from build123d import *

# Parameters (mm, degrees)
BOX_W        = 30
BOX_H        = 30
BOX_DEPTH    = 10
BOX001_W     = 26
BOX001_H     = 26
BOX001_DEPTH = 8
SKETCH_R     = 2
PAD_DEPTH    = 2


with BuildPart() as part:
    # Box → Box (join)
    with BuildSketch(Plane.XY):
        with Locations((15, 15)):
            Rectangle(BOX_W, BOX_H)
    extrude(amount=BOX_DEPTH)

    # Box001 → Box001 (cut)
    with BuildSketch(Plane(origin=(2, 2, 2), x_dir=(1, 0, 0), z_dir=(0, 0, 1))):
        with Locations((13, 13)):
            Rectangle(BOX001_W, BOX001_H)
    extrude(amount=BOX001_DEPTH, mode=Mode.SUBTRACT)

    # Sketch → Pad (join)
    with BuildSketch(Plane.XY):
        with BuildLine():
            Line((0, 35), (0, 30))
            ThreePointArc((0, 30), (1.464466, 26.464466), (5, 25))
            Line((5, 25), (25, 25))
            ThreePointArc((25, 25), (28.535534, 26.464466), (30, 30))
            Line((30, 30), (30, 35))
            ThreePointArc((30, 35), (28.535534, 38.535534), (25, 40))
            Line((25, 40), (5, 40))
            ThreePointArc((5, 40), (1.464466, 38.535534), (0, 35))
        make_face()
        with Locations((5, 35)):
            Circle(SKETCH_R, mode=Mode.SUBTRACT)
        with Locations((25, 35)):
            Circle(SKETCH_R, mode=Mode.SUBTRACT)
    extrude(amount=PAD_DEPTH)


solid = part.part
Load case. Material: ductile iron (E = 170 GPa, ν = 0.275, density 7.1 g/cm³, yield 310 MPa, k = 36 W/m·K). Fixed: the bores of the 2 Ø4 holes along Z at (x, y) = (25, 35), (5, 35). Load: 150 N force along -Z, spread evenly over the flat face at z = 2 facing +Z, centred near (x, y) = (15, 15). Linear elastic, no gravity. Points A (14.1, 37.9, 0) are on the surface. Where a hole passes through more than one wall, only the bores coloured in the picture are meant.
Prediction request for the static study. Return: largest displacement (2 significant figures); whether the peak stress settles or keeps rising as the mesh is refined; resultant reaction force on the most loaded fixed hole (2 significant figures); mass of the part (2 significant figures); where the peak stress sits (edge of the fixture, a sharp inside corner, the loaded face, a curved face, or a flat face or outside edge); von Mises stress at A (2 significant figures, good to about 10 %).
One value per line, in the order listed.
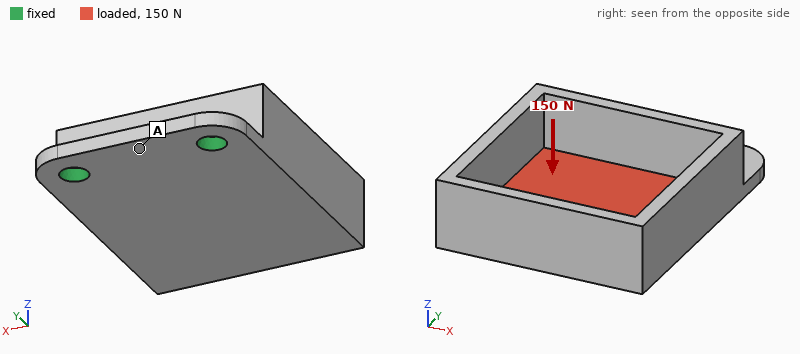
0.14 mm
keeps rising
82 N
29 g
edge of the fixture
20 MPa
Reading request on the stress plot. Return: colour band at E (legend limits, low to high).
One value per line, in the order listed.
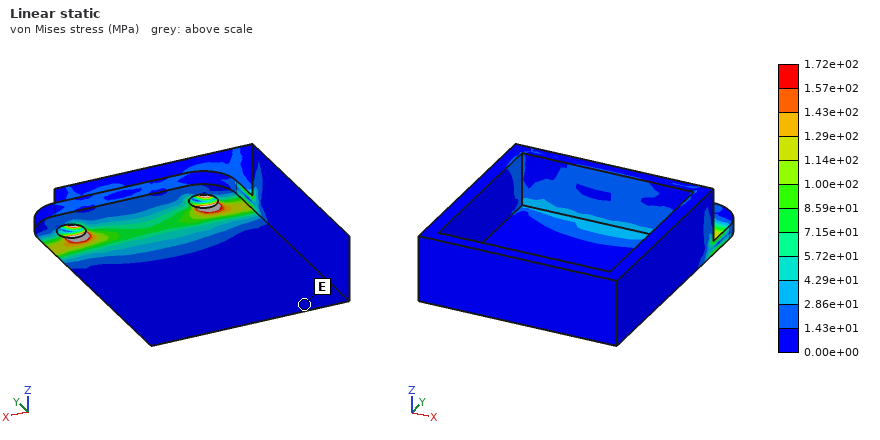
0.00e+00 to 1.43e+01 MPa
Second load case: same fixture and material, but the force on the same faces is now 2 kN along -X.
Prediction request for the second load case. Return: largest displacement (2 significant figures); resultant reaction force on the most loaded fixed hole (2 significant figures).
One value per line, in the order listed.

56 µm
2.0 kN
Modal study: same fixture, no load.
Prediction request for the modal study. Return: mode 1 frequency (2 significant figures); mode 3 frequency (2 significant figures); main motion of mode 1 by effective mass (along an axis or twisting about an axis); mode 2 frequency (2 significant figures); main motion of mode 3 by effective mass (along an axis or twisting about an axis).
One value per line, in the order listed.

1200 Hz
9300 Hz
along Z
3100 Hz
along X
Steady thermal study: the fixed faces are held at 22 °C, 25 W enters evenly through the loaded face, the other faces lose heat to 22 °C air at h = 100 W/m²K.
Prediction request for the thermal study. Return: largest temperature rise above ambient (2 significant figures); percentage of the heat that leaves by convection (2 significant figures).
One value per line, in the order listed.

76 K
62 %
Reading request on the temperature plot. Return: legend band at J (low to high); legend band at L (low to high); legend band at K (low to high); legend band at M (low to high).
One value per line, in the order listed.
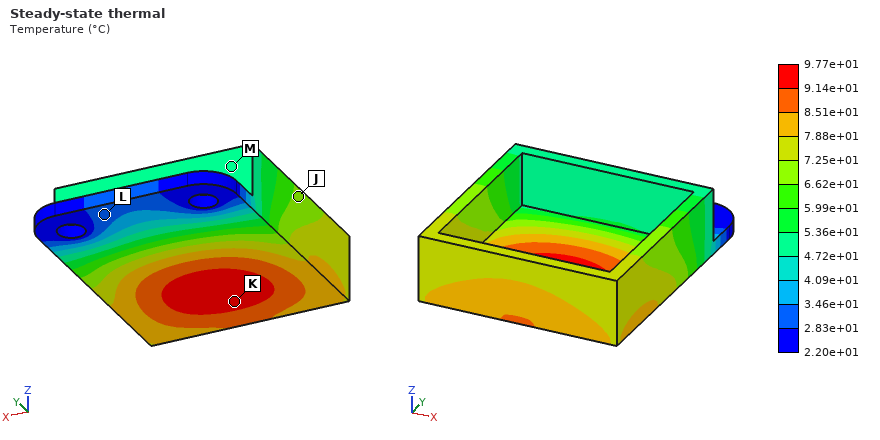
6.62e+01 to 7.25e+01 °C
2.83e+01 to 3.46e+01 °C
9.14e+01 to 9.77e+01 °C
4.72e+01 to 5.36e+01 °C
